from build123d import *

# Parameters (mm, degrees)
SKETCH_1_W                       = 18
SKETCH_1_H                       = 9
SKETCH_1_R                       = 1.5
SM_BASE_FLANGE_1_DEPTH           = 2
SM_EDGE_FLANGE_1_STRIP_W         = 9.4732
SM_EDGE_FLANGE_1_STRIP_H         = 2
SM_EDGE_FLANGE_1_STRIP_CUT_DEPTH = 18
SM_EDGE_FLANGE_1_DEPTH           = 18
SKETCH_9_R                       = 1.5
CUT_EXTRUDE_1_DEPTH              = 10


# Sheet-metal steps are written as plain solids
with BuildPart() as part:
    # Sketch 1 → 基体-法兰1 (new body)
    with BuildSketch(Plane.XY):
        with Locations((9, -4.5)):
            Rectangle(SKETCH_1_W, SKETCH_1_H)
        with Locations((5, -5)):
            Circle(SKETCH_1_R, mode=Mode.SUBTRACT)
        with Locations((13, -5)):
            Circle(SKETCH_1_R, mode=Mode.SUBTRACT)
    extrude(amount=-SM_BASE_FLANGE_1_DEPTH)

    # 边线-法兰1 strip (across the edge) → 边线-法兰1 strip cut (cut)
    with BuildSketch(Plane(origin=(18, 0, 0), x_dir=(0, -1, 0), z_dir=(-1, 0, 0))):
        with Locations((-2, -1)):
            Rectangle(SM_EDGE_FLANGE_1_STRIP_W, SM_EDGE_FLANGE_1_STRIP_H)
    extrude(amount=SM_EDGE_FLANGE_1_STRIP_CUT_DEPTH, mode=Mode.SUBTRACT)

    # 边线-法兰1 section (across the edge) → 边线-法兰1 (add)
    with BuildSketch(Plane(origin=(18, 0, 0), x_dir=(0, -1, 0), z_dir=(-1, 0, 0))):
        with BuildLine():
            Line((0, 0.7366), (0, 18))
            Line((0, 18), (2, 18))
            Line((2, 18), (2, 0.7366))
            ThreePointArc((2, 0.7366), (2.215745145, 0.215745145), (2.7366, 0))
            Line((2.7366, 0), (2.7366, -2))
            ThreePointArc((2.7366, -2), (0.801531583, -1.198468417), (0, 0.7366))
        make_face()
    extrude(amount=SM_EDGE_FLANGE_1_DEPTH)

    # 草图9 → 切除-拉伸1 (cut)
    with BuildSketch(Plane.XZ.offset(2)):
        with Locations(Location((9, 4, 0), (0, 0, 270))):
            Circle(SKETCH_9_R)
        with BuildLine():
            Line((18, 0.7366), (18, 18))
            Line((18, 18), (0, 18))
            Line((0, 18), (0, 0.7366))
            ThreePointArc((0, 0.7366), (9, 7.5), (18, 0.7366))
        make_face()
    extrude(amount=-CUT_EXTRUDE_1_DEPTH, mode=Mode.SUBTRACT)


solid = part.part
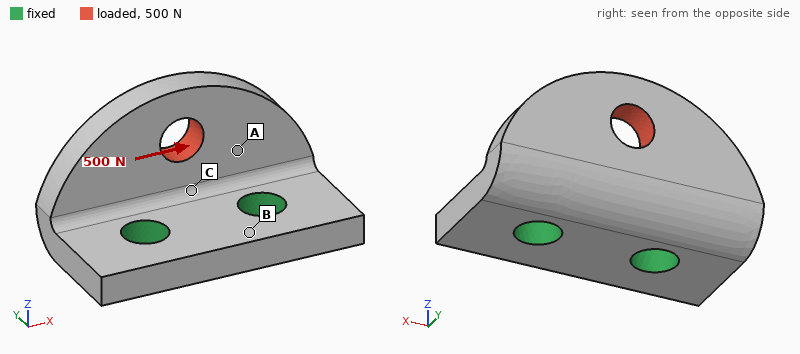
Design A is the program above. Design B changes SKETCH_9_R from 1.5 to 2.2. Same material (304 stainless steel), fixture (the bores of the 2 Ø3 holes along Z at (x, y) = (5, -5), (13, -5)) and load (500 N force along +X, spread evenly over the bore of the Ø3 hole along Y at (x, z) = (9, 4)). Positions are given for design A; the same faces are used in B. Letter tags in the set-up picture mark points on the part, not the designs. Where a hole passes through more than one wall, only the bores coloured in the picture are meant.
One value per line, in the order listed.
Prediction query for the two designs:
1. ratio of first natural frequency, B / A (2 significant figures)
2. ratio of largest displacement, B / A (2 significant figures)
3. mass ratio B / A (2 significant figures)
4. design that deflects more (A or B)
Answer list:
1.0
1.2
0.96
B
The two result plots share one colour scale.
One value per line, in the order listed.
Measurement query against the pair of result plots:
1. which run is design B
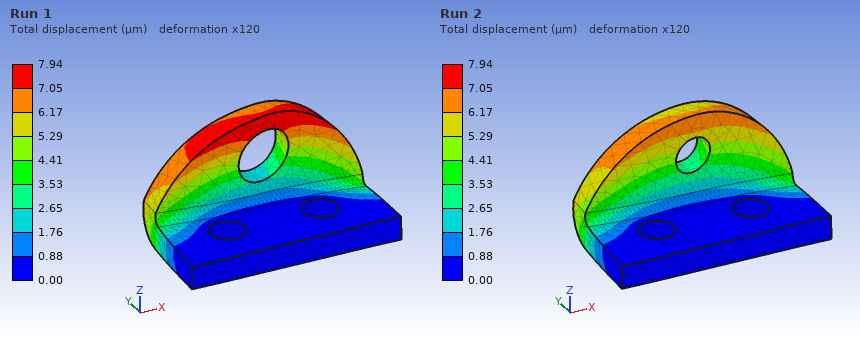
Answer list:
Run 1
